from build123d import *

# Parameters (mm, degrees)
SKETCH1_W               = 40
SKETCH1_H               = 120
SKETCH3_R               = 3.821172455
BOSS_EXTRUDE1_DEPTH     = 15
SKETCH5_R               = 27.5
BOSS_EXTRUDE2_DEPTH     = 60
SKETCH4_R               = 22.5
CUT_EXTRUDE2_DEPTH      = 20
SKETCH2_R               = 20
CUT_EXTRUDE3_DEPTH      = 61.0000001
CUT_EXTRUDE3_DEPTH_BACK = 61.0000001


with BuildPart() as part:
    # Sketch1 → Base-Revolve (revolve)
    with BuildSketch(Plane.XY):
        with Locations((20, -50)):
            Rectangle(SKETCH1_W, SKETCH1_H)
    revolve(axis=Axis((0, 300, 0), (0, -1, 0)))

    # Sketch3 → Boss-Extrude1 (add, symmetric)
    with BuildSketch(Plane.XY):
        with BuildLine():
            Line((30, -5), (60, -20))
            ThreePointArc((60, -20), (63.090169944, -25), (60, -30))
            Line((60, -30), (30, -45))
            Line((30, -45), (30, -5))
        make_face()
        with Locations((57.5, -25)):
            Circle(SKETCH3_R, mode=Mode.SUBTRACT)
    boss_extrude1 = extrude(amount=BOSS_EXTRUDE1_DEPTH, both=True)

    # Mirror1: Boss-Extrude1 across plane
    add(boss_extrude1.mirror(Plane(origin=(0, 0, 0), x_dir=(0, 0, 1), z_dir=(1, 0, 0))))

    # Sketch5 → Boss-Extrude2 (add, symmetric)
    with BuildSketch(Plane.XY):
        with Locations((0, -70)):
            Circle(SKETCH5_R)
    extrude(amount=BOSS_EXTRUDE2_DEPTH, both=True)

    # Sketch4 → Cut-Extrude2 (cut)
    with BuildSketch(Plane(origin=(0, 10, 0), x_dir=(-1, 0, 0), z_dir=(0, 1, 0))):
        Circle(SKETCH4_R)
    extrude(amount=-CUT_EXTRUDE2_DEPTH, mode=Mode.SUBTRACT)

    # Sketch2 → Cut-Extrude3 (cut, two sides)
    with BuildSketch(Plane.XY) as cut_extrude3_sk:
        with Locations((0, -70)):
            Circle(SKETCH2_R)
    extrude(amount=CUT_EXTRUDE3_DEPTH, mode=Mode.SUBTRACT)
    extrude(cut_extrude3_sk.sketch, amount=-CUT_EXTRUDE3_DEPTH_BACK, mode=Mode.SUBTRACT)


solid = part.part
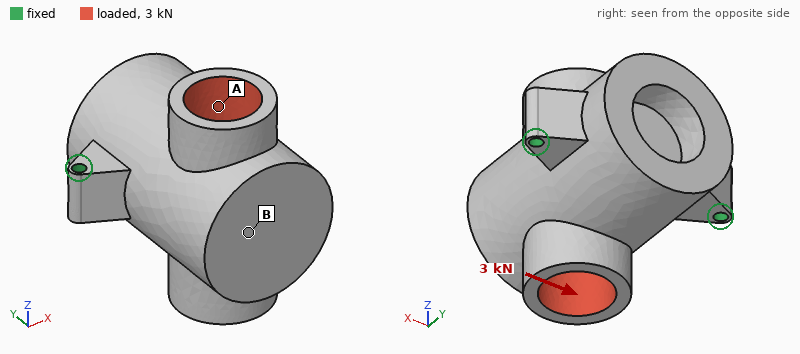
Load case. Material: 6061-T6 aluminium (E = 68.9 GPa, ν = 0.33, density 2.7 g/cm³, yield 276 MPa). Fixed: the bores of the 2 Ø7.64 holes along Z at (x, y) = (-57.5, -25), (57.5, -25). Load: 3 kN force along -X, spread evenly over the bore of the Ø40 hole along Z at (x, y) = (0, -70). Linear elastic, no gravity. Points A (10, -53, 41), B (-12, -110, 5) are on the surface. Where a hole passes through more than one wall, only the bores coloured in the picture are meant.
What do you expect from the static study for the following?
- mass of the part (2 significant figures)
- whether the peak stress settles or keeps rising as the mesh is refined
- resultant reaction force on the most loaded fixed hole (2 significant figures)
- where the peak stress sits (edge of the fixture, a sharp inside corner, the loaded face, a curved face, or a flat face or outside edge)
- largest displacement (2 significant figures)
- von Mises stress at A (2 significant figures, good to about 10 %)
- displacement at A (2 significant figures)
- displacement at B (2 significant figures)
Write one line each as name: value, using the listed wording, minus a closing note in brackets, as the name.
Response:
mass of the part: 1.5 kg
whether the peak stress settles or keeps rising as the mesh is refined: keeps rising
resultant reaction force on the most loaded fixed hole: 2.0 kN
where the peak stress sits: edge of the fixture
largest displacement: 8.7 µm
von Mises stress at A: 2.4 MPa
displacement at A: 2.9 µm
displacement at B: 8.2 µm
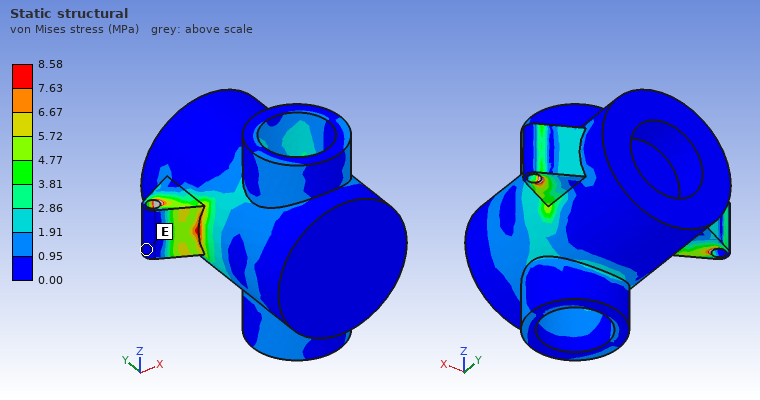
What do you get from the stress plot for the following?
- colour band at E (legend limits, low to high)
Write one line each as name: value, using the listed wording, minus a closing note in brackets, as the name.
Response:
colour band at E: 0.00 to 0.95 MPa
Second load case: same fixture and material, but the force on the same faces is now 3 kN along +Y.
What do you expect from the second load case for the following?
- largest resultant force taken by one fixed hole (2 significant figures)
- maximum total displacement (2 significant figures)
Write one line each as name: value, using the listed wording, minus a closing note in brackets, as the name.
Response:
largest resultant force taken by one fixed hole: 1.5 kN
maximum total displacement: 4.8 µm
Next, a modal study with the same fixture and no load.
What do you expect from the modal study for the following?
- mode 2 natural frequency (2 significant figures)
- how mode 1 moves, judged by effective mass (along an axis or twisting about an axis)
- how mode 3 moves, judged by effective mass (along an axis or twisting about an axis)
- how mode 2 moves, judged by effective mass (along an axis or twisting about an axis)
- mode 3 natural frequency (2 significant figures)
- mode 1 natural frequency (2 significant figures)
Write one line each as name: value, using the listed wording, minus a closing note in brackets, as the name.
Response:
mode 2 natural frequency: 3400 Hz
how mode 1 moves, judged by effective mass: along Z
how mode 3 moves, judged by effective mass: along Y
how mode 2 moves, judged by effective mass: along X
mode 3 natural frequency: 3800 Hz
mode 1 natural frequency: 1000 Hz
